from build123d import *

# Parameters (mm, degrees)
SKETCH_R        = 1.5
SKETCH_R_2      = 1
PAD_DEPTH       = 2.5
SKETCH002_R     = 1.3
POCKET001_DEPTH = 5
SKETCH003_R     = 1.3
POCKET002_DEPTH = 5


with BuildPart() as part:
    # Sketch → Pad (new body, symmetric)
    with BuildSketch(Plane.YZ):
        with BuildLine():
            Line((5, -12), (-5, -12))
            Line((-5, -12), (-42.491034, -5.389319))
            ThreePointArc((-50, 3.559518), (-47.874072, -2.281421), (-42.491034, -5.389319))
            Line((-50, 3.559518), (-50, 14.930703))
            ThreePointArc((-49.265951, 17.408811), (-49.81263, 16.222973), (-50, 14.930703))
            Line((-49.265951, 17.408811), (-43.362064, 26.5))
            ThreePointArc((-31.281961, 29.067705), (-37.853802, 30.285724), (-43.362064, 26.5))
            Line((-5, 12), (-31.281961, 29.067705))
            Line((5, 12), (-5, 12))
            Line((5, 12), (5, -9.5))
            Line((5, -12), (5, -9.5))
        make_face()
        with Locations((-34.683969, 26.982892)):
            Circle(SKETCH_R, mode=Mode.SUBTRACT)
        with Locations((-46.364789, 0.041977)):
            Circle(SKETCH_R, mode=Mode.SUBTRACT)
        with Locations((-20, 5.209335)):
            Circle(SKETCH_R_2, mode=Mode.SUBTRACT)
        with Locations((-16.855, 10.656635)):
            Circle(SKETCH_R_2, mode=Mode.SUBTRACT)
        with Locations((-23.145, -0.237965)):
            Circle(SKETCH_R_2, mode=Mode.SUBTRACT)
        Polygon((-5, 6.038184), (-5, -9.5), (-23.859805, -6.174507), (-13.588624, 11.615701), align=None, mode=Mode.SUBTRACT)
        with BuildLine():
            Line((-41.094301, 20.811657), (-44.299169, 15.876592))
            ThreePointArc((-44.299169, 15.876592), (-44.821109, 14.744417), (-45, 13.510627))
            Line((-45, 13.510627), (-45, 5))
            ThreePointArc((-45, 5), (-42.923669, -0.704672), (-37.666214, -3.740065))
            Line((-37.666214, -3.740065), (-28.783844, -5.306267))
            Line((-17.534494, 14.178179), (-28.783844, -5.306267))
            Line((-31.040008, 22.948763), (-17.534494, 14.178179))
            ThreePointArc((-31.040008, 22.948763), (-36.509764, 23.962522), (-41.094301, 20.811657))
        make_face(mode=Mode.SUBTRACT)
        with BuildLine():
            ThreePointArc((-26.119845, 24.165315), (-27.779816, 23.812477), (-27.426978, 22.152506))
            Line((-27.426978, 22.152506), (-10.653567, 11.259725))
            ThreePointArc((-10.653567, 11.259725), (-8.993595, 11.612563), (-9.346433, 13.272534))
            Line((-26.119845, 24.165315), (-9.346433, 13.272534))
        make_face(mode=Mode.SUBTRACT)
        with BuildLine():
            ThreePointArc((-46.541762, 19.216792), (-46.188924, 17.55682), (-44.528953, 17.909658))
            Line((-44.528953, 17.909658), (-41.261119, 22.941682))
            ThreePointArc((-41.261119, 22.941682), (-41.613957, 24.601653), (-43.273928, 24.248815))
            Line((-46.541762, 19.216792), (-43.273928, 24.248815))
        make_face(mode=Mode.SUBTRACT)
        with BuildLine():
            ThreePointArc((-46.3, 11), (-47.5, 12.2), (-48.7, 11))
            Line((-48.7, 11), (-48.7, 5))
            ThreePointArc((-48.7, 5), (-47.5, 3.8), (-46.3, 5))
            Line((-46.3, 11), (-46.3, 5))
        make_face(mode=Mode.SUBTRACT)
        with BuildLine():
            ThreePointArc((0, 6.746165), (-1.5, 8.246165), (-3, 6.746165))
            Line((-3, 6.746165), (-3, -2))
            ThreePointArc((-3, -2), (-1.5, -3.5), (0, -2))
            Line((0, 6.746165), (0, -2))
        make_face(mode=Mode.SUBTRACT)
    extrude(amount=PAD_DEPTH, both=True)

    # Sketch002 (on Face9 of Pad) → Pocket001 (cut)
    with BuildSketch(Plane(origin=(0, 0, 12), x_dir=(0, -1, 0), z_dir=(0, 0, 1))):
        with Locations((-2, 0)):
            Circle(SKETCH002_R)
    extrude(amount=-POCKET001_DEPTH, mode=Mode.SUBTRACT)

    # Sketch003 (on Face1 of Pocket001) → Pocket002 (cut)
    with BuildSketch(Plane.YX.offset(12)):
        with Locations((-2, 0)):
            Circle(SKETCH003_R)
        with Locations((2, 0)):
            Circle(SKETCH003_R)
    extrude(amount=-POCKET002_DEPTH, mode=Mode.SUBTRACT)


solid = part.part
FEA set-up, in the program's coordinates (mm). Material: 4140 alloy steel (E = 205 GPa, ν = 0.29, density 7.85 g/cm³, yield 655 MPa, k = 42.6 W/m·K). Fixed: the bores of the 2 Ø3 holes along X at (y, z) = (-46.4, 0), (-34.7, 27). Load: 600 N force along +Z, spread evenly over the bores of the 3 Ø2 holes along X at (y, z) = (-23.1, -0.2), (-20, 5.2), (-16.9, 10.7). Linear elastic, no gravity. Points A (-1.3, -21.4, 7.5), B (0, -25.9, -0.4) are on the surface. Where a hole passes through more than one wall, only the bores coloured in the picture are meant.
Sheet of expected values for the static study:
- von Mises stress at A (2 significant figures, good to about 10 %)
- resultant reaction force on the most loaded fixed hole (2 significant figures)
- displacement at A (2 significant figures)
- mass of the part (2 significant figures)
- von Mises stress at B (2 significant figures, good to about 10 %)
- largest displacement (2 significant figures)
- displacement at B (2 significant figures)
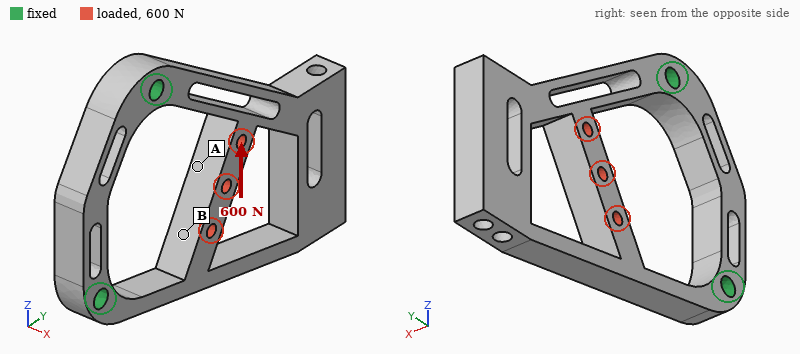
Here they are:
64 MPa
400 N
0.11 mm
26 g
150 MPa
0.11 mm
0.10 mm
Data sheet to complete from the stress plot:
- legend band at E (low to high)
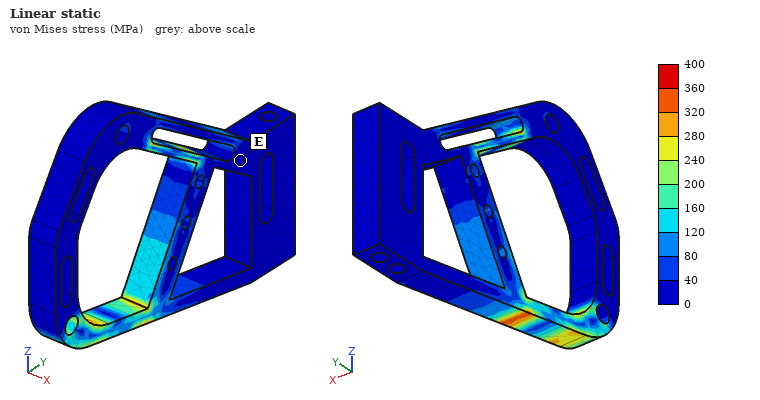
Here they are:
0 to 40 MPa
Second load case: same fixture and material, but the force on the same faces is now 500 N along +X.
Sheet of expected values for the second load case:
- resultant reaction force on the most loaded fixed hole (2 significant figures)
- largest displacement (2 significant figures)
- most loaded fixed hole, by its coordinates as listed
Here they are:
280 N
0.38 mm
(-34.7, 27)
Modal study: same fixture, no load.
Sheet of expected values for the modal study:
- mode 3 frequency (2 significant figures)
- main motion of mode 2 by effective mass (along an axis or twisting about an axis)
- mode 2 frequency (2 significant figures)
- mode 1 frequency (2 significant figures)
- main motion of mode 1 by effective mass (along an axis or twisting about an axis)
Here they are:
4300 Hz
along Z
3100 Hz
1200 Hz
along X
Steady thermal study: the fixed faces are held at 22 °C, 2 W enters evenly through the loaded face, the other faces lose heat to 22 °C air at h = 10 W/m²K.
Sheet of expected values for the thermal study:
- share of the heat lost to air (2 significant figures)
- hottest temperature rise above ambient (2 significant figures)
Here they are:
28 %
35 K
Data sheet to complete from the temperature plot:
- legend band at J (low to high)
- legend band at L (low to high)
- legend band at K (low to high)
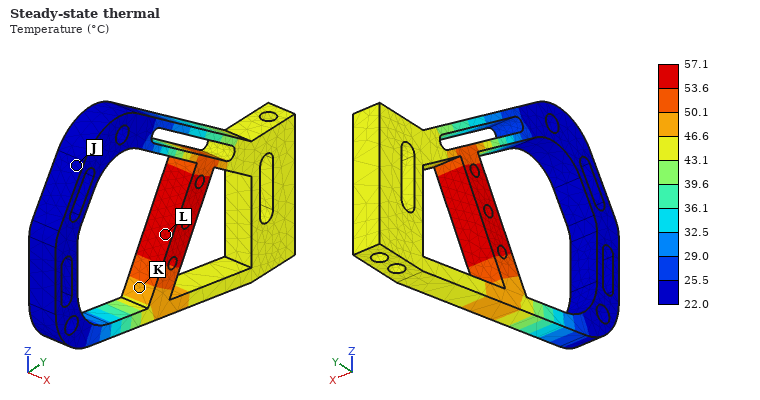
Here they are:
22.0 to 25.5 °C
53.6 to 57.1 °C
46.6 to 50.1 °C
